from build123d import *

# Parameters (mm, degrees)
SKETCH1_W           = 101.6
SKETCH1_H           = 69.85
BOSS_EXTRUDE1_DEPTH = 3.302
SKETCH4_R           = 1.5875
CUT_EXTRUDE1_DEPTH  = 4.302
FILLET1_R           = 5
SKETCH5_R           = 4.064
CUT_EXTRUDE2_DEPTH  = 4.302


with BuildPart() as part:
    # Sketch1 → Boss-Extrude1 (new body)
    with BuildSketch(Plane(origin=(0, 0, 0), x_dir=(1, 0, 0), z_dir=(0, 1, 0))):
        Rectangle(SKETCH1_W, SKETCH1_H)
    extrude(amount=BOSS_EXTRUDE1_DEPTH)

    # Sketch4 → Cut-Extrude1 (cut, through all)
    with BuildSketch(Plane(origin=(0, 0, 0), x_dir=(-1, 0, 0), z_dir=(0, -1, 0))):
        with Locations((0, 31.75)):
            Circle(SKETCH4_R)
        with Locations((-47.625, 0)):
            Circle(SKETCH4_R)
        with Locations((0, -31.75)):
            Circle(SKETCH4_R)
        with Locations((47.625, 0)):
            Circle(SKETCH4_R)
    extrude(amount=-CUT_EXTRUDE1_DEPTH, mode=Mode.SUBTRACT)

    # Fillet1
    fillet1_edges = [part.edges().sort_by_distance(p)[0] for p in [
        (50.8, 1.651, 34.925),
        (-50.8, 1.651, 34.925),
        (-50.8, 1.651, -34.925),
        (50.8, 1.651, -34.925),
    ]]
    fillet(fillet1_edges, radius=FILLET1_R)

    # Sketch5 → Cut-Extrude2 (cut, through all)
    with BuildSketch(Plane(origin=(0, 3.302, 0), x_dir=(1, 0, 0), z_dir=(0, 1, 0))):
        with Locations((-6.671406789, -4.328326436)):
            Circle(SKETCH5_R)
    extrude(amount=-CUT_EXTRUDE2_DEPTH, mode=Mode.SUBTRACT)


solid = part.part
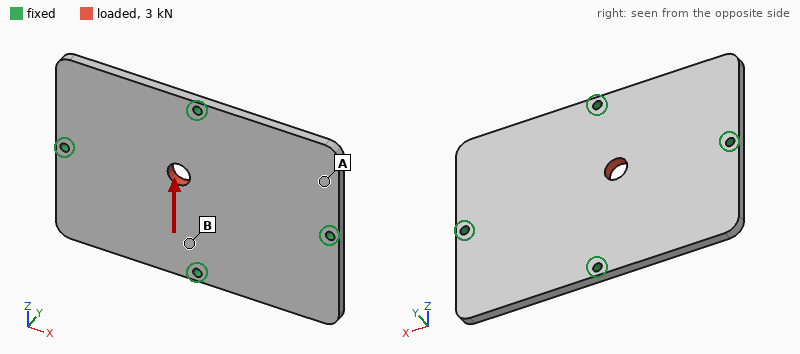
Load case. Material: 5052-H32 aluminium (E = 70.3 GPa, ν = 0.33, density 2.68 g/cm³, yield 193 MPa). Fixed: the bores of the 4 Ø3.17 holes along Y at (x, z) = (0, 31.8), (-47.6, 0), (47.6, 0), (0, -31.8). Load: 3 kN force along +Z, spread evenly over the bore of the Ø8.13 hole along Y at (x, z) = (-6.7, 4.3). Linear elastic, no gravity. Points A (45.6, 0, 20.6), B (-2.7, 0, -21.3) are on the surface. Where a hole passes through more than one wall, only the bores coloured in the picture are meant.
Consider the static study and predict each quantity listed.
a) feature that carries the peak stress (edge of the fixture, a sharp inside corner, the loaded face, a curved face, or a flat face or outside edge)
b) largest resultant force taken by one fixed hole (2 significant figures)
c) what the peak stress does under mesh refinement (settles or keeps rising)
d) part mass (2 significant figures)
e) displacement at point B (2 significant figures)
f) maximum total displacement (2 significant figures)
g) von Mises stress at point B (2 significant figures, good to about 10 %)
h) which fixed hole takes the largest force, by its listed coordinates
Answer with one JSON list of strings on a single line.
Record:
["edge of the fixture", "1.2 kN", "keeps rising", "62 g", "4.2 µm", "12 µm", "22 MPa", "(0, 31.8)"]
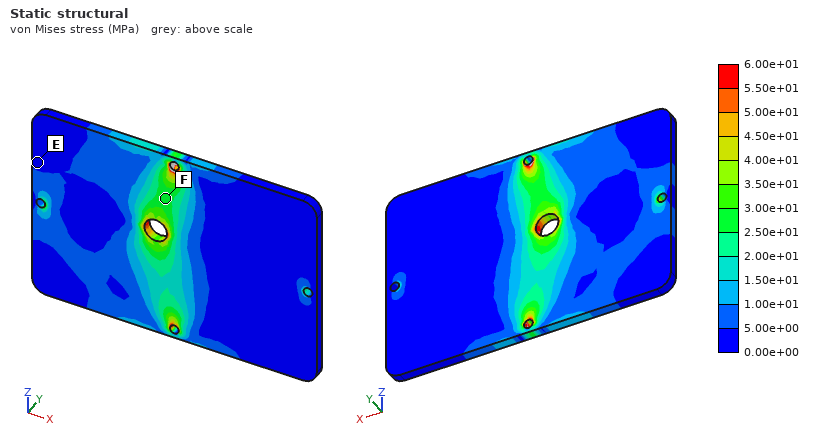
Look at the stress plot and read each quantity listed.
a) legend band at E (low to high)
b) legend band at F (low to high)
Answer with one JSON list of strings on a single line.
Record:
["0.00e+00 to 5.00e+00 MPa", "2.50e+01 to 3.00e+01 MPa"]
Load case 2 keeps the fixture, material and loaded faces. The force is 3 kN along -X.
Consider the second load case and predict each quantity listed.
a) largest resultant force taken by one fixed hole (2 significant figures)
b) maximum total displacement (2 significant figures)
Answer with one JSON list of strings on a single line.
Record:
["910 N", "11 µm"]
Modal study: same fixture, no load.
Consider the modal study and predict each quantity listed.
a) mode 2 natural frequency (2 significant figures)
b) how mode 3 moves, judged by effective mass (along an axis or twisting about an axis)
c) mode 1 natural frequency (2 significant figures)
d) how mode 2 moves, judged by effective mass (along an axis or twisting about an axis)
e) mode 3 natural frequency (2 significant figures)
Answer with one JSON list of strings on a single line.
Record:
["3000 Hz", "twisting about Z", "2900 Hz", "twisting about X", "3200 Hz"]
